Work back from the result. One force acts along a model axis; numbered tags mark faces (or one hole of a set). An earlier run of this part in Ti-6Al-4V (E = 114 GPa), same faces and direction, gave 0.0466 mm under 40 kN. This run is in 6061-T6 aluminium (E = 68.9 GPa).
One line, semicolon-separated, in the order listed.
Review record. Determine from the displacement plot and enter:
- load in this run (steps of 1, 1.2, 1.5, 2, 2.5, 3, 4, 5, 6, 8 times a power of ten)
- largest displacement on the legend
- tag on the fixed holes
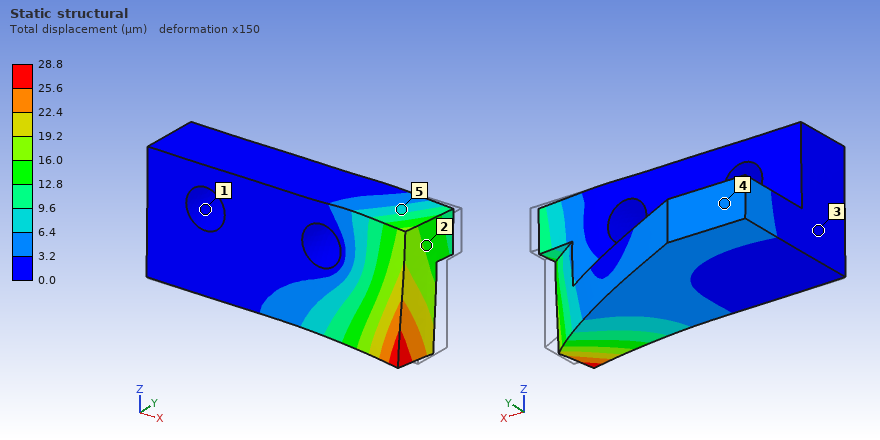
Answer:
15 kN; 28.8 µm; 1
